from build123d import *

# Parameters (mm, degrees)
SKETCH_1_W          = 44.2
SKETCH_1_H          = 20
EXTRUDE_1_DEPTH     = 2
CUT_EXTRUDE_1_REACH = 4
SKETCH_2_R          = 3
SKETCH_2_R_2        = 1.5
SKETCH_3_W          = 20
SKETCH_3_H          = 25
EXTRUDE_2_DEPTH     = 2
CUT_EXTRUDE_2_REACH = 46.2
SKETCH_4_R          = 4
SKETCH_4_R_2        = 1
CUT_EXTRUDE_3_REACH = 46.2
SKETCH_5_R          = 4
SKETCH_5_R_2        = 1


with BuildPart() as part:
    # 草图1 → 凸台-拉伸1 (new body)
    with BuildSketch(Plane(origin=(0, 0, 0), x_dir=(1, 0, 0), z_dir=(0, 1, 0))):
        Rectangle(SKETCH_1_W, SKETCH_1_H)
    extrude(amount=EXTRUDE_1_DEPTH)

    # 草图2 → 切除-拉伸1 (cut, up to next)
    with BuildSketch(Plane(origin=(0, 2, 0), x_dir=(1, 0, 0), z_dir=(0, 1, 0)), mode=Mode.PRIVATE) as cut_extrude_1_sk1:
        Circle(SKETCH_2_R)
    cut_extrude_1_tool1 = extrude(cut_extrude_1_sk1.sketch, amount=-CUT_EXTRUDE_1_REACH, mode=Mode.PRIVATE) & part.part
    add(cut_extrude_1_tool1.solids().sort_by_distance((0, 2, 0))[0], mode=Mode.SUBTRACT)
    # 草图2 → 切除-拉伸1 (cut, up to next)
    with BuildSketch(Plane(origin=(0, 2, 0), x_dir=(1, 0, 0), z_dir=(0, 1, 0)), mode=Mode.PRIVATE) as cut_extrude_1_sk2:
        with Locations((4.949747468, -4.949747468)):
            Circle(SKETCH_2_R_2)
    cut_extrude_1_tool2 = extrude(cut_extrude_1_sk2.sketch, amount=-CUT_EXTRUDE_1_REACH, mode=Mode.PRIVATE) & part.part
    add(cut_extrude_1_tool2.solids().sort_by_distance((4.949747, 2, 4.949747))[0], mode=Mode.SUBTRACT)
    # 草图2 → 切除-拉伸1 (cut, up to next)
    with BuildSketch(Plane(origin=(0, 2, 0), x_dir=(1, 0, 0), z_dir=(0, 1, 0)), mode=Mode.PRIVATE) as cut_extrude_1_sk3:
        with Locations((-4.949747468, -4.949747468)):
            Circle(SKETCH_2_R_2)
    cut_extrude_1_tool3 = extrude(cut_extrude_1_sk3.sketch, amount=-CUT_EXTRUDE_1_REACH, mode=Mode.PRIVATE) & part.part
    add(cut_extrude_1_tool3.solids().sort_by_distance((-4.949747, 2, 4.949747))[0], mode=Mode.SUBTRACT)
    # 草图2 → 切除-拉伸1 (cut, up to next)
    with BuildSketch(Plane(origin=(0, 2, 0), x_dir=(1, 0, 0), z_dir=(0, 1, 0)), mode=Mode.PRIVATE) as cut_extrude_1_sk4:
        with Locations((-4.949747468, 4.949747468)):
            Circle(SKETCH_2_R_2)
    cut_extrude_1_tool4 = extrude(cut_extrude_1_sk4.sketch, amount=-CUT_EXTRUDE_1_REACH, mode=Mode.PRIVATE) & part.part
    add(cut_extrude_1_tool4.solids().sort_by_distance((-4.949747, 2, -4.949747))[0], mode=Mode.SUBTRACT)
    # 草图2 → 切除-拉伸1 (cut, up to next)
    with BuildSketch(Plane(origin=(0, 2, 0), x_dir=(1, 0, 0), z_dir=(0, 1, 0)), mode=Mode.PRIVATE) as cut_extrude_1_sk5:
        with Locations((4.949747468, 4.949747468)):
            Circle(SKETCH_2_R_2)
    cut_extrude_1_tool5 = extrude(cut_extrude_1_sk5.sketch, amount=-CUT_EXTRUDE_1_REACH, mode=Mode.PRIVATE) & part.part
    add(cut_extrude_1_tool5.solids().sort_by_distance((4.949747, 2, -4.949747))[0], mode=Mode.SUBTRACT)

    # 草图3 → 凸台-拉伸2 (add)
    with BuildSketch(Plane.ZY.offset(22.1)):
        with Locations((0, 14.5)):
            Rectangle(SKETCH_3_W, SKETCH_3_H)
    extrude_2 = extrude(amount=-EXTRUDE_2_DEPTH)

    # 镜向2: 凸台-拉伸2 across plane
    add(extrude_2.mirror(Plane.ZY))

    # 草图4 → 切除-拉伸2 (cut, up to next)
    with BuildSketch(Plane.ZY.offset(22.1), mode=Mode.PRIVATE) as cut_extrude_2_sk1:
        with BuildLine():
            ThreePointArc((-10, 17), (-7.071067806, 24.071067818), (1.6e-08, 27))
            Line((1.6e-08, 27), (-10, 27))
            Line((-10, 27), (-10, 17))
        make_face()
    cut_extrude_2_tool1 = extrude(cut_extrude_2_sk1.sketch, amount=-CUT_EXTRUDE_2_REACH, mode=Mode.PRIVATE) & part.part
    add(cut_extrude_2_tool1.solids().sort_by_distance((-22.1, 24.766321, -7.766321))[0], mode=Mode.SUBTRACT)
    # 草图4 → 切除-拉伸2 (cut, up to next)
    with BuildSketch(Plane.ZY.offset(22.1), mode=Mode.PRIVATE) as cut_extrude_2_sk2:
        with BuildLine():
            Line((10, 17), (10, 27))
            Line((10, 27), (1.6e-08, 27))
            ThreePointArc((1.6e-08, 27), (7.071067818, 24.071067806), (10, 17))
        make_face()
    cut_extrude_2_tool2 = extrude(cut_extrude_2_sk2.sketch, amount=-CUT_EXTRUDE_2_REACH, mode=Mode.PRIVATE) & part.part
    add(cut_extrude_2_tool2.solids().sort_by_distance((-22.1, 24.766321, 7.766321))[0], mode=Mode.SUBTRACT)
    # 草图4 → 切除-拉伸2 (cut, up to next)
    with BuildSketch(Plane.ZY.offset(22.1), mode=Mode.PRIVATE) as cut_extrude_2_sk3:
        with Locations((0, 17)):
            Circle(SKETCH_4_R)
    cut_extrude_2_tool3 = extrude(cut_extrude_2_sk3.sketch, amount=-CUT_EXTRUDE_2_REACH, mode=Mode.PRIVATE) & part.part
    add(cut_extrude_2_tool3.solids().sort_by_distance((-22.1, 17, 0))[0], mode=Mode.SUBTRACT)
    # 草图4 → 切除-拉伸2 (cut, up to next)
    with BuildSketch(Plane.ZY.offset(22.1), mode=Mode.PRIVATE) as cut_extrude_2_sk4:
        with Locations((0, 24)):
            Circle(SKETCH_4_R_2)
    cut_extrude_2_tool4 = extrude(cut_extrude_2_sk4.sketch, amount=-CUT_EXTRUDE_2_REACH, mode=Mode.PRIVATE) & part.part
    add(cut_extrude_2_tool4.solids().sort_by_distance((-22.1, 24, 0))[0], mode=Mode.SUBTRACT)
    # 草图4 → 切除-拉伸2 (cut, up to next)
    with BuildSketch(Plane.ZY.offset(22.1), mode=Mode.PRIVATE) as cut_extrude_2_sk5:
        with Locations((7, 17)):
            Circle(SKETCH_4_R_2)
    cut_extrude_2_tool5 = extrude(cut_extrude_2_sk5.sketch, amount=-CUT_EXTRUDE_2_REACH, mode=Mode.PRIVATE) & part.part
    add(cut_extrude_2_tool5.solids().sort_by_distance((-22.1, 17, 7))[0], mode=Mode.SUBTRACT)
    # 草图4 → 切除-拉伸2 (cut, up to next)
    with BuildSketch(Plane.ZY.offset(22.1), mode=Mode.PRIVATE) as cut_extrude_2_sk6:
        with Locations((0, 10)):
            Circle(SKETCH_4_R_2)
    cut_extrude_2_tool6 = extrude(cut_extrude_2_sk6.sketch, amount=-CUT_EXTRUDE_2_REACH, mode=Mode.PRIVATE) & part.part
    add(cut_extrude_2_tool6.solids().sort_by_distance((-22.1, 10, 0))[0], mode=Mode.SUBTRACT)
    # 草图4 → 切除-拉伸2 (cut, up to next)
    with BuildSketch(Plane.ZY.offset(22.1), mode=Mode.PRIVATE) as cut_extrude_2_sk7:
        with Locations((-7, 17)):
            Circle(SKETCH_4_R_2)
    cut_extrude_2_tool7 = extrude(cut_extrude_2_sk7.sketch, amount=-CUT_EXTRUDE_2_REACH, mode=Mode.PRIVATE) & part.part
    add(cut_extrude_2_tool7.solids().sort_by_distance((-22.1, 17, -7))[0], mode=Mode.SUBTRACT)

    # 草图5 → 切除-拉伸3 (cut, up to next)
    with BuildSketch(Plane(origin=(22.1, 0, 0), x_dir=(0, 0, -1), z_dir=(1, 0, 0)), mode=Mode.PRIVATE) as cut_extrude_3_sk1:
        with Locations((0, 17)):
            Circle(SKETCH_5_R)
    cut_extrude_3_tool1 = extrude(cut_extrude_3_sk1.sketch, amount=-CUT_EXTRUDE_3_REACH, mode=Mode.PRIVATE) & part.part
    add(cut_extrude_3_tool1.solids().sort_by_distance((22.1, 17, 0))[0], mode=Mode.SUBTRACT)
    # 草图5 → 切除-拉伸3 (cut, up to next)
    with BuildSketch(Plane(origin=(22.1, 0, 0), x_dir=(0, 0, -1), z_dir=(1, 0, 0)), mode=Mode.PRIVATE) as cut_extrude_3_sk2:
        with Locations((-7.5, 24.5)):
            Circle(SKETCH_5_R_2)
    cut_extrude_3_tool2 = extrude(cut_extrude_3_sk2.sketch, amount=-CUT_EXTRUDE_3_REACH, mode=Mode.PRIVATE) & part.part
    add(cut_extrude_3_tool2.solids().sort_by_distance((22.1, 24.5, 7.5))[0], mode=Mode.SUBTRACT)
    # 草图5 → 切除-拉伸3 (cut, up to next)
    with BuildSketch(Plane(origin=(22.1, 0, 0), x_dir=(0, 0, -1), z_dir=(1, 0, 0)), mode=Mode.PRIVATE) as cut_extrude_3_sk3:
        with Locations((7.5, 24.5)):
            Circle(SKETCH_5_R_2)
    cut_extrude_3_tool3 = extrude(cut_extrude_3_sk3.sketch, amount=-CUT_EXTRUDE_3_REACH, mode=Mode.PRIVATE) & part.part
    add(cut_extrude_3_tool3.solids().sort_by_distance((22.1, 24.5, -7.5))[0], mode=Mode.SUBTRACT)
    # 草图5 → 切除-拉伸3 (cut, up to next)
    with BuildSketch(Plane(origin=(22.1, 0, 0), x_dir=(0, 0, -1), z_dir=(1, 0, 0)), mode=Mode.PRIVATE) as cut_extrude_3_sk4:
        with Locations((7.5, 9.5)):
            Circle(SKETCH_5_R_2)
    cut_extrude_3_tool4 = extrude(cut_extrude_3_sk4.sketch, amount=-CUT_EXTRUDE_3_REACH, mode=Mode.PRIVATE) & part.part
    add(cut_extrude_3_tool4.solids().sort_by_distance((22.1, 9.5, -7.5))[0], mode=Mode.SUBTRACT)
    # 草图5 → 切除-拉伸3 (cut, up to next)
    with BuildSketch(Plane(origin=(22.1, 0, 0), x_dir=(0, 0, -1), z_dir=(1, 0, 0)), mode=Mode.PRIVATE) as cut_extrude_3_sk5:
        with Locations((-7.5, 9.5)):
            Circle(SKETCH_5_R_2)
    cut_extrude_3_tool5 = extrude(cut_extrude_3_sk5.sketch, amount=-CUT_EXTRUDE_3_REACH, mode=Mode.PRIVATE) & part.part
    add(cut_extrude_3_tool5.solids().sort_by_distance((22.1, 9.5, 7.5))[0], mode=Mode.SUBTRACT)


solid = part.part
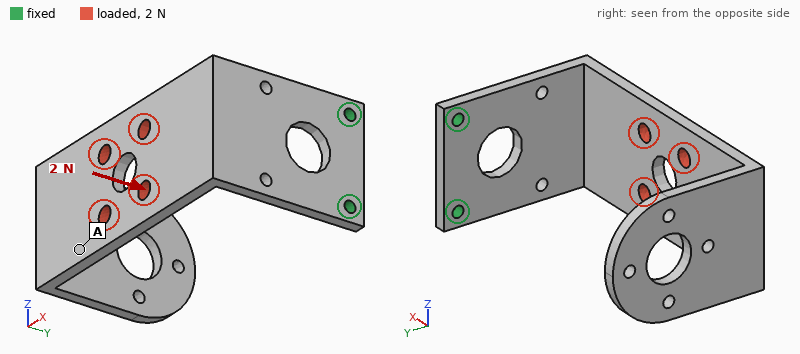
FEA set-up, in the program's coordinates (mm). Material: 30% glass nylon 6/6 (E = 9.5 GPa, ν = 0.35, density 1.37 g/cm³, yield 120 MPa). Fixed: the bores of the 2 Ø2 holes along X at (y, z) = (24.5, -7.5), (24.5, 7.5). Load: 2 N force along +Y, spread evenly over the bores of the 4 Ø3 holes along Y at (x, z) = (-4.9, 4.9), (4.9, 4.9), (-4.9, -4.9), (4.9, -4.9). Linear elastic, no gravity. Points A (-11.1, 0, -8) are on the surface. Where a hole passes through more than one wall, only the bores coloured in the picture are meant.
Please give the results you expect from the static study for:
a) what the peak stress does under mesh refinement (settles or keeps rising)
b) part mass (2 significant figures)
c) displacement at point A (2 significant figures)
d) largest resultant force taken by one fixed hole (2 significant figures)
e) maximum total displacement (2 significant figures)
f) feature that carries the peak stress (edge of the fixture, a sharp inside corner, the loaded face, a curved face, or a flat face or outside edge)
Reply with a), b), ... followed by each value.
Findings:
a) keeps rising
b) 4.5 g
c) 0.42 mm
d) 1.0 N
e) 0.59 mm
f) edge of the fixture
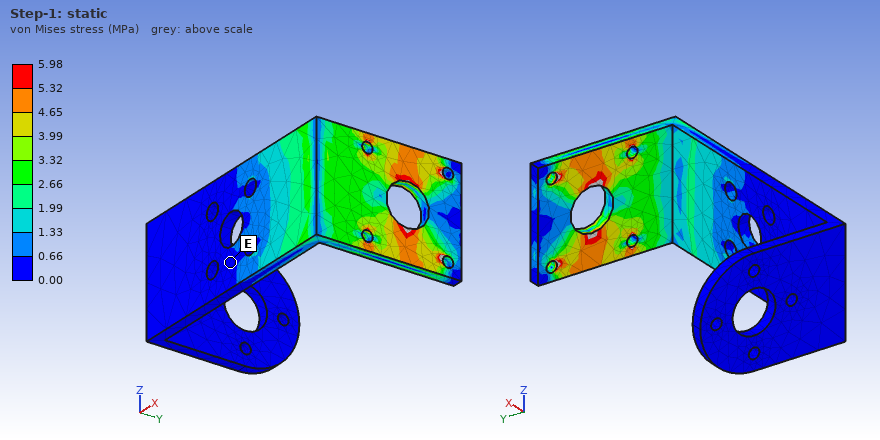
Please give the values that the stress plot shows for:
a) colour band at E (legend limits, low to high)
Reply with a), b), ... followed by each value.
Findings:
a) 0.00 to 0.66 MPa
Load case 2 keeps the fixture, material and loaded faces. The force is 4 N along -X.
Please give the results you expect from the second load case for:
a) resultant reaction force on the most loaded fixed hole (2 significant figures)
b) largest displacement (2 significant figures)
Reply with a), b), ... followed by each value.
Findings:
a) 2.0 N
b) 0.54 mm
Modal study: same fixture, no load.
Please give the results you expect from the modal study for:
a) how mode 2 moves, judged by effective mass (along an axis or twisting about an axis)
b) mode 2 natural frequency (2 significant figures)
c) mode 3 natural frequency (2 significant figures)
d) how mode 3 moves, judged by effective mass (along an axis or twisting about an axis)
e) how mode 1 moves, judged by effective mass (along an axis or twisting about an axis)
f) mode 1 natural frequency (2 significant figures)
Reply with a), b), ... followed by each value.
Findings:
a) along Z
b) 250 Hz
c) 470 Hz
d) along X
e) along Y
f) 150 Hz
